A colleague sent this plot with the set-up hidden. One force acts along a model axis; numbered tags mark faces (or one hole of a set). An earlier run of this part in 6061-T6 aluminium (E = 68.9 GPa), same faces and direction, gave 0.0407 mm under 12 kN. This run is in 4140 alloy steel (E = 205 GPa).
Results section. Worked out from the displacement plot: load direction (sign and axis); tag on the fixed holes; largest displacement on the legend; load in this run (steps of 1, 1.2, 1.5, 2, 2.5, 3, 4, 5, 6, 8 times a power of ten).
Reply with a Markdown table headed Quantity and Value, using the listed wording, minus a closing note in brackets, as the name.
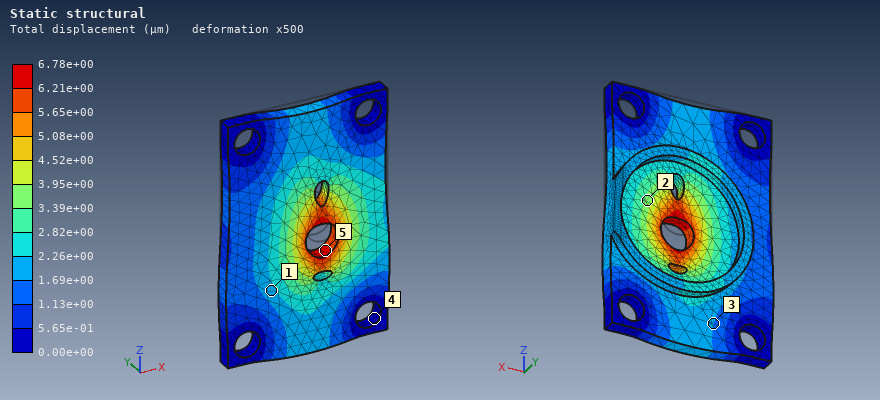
| Quantity | Value |
|---|---|
| load direction | -Z |
| tag on the fixed holes | 4 |
| largest displacement on the legend | 6.78e+00 µm |
| load in this run | 6 kN |
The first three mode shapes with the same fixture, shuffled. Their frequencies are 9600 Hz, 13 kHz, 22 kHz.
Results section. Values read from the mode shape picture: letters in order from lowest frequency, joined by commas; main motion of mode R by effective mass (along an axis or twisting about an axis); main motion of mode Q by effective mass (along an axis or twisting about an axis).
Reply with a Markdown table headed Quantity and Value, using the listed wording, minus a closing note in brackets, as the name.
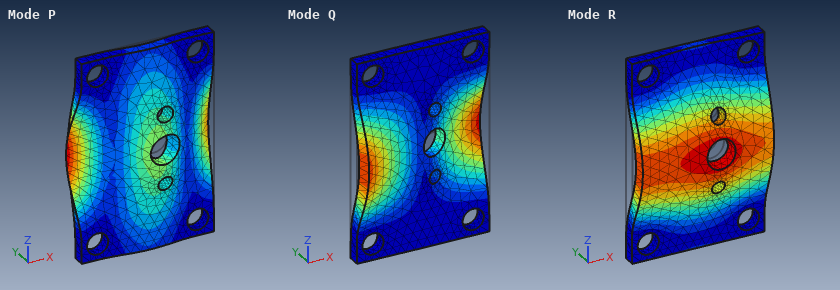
| Quantity | Value |
|---|---|
| letters in order from lowest frequency, joined by commas | R, Q, P |
| main motion of mode R by effective mass | along Y |
| main motion of mode Q by effective mass | twisting about Z |
